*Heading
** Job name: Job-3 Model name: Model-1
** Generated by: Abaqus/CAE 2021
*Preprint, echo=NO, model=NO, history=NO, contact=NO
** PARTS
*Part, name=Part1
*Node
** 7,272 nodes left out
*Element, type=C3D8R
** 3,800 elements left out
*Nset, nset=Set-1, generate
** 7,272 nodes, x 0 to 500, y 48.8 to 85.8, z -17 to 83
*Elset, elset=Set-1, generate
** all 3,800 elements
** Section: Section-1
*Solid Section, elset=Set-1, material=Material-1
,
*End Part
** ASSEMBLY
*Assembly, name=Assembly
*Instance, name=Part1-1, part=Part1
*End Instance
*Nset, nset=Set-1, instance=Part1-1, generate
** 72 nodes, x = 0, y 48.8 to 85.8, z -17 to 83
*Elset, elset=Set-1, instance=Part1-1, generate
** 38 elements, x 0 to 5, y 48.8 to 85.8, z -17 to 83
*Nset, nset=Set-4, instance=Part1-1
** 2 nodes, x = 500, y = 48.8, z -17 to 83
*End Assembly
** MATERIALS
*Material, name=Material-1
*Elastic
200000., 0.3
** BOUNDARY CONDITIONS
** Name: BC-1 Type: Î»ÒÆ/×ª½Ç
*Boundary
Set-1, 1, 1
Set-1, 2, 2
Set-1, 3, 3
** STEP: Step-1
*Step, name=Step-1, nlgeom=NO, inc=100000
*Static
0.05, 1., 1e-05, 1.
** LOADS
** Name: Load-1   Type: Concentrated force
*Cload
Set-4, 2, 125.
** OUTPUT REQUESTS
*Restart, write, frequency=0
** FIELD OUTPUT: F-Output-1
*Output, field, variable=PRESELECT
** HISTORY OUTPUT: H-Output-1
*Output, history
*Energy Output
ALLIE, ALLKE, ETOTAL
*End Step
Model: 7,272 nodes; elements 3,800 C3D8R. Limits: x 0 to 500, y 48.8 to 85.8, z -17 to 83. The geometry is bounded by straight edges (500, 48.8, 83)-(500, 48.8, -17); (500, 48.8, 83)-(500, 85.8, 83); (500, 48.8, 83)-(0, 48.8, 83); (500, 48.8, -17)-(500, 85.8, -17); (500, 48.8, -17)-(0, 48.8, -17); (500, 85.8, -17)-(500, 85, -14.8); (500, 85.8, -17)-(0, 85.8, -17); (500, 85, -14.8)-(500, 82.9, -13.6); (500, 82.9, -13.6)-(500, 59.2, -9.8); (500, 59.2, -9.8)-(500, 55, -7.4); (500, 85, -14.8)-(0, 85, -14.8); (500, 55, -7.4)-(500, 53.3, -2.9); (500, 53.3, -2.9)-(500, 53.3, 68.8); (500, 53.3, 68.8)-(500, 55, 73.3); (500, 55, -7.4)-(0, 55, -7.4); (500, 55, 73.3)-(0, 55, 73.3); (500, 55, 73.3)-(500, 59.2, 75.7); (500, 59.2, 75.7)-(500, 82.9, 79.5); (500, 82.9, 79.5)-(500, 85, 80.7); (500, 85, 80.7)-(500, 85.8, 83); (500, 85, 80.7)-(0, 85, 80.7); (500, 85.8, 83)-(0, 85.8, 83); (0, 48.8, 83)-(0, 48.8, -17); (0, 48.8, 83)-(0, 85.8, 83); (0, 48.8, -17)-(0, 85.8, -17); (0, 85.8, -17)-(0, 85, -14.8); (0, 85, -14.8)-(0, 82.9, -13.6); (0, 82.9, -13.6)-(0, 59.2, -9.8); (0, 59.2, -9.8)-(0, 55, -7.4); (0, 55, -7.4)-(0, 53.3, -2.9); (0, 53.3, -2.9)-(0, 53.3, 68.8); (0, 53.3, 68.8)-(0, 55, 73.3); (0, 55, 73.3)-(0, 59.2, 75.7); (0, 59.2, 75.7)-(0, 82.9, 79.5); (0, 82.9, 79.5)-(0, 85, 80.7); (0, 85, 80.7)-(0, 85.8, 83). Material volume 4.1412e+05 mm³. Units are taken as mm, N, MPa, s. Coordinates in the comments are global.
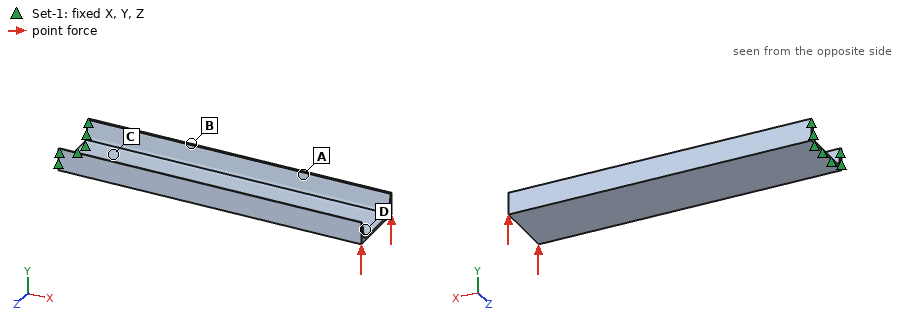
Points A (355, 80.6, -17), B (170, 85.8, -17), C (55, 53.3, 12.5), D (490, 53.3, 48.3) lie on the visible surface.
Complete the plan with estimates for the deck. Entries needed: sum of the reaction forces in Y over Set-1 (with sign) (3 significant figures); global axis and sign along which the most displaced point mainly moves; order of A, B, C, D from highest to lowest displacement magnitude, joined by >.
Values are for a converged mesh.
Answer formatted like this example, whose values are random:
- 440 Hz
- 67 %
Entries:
- -250 N
- +Y
- D > A > B > C
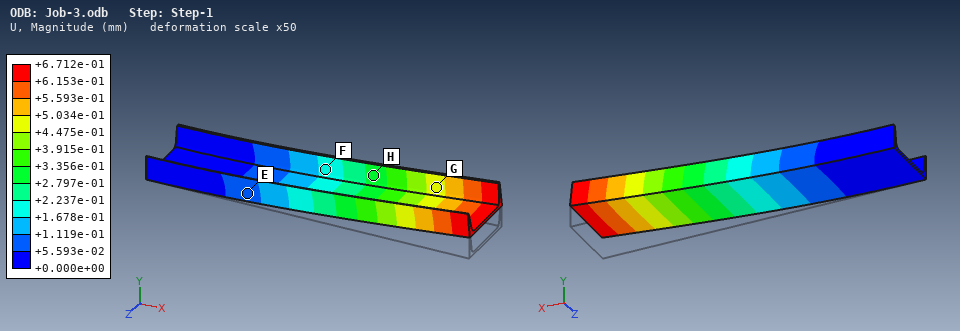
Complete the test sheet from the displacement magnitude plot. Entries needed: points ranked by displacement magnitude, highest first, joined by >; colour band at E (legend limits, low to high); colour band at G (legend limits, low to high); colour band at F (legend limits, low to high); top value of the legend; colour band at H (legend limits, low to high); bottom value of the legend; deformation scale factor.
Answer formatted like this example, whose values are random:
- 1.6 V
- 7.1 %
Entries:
- G > H > F > E
- +5.593e-02 to +1.119e-01 mm
- +4.475e-01 to +5.034e-01 mm
- +1.678e-01 to +2.237e-01 mm
- +6.712e-01 mm
- +2.797e-01 to +3.356e-01 mm
- +0.000e+00 mm
- 50
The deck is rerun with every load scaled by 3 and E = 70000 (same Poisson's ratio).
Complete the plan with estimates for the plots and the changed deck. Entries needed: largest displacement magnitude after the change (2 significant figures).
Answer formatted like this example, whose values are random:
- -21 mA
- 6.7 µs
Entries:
- 5.8 mm
